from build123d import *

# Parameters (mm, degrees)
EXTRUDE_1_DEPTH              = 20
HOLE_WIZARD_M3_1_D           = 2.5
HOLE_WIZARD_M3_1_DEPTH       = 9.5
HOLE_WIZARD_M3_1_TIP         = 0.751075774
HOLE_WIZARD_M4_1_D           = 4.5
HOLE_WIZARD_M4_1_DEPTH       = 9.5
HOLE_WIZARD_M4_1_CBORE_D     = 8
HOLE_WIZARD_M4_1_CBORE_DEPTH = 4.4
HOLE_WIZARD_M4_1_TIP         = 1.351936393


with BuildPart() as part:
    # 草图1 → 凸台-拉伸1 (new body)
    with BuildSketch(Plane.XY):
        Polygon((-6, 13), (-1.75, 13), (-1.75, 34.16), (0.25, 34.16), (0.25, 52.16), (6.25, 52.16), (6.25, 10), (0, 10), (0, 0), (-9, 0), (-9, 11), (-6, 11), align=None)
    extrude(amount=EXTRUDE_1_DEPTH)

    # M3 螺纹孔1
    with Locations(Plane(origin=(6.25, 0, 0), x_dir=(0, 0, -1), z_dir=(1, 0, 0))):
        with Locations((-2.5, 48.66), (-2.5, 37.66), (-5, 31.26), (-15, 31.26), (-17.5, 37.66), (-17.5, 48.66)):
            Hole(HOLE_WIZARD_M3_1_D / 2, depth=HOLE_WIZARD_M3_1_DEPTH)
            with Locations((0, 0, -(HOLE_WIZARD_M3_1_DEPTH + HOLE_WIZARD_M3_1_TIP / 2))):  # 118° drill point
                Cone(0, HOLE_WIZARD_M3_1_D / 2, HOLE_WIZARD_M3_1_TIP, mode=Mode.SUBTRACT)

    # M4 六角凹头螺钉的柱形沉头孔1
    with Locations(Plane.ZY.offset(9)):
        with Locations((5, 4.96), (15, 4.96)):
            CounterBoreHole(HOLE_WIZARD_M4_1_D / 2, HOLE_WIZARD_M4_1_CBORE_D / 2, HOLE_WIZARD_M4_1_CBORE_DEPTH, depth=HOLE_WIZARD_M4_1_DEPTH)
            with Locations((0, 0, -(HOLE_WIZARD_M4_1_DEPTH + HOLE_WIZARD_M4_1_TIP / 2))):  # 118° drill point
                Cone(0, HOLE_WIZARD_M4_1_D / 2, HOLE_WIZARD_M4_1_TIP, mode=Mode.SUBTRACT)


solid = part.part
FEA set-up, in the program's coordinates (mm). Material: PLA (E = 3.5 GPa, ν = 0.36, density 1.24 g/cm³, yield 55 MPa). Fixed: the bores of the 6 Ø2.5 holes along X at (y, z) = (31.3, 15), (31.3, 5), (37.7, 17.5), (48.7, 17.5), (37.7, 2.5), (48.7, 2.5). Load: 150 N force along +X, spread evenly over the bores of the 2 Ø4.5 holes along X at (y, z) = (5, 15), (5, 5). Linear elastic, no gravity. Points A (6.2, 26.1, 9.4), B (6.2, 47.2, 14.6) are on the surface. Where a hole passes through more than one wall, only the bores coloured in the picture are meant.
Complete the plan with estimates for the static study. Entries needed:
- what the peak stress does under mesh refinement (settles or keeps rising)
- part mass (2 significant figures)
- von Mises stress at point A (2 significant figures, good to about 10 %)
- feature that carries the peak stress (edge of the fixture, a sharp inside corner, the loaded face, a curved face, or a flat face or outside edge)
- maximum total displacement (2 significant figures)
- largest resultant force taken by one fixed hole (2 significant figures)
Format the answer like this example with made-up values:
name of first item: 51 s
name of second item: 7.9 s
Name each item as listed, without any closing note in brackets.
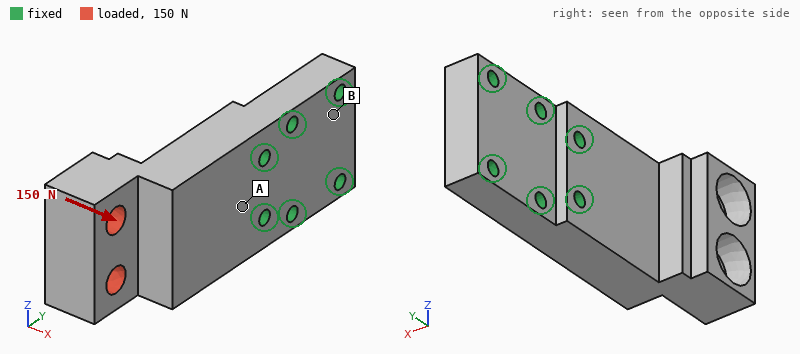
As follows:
what the peak stress does under mesh refinement: keeps rising
part mass: 9.1 g
von Mises stress at point A: 13 MPa
feature that carries the peak stress: edge of the fixture
maximum total displacement: 0.59 mm
largest resultant force taken by one fixed hole: 120 N
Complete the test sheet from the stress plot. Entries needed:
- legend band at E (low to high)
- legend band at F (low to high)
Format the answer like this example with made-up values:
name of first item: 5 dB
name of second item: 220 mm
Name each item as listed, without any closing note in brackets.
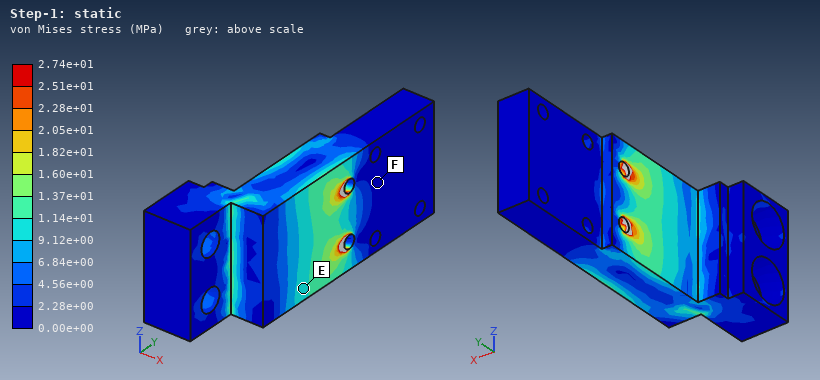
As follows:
legend band at E: 9.12e+00 to 1.14e+01 MPa
legend band at F: 0.00e+00 to 2.28e+00 MPa
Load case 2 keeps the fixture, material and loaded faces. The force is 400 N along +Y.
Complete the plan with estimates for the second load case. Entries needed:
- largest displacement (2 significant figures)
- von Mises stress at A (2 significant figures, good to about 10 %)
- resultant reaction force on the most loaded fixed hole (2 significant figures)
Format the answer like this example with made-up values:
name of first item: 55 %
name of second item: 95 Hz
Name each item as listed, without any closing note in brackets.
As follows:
largest displacement: 0.36 mm
von Mises stress at A: 5.4 MPa
resultant reaction force on the most loaded fixed hole: 180 N
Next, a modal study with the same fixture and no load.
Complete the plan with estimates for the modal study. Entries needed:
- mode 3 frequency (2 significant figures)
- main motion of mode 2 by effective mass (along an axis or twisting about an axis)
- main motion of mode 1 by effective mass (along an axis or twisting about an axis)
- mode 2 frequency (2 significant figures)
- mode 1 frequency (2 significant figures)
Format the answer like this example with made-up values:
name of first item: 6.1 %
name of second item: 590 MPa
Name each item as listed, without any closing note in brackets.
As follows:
mode 3 frequency: 5300 Hz
main motion of mode 2 by effective mass: along Z
main motion of mode 1 by effective mass: along X
mode 2 frequency: 3700 Hz
mode 1 frequency: 2000 Hz
